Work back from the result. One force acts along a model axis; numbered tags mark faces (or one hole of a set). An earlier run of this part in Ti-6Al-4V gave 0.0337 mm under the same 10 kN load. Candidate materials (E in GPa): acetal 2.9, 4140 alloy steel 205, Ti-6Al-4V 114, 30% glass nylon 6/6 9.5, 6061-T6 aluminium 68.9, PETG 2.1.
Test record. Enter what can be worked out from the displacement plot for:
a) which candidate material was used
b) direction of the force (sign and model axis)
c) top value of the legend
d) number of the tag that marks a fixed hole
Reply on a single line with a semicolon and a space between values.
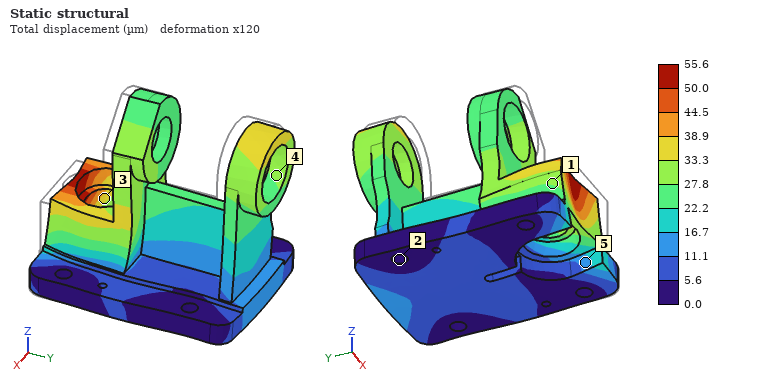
6061-T6 aluminium; +Y; 55.6 µm; 2
